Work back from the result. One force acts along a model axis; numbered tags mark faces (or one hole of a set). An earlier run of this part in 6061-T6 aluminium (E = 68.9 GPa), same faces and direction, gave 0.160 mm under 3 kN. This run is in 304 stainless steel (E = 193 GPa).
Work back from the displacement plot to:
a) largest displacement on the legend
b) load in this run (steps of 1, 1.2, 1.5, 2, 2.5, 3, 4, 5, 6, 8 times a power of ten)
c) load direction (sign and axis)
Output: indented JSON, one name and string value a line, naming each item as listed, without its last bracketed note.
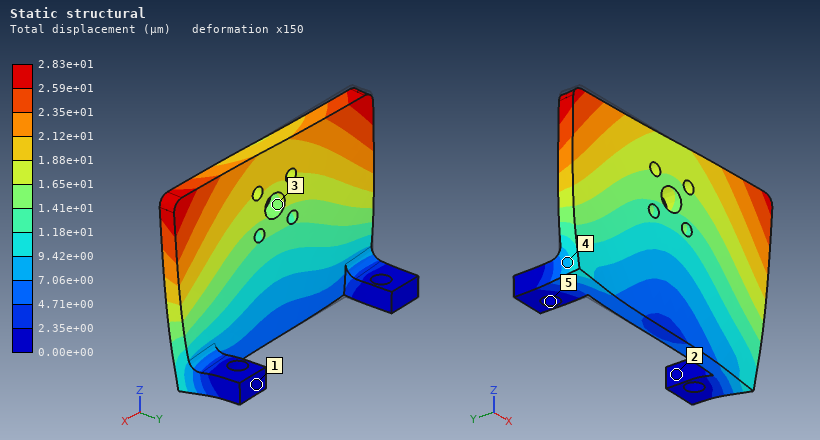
{
  "largest displacement on the legend": "2.83e+01 µm",
  "load in this run": "1.5 kN",
  "load direction": "+X"
}
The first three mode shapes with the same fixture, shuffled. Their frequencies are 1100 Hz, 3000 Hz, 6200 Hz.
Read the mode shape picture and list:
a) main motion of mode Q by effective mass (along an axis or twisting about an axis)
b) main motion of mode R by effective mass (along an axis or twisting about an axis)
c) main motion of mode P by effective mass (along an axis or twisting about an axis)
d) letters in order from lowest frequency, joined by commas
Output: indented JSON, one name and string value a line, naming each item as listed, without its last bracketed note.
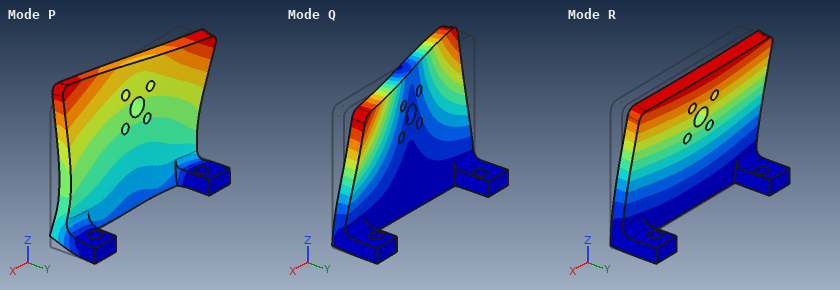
{
  "main motion of mode Q by effective mass": "twisting about Z",
  "main motion of mode R by effective mass": "along Y",
  "main motion of mode P by effective mass": "along X",
  "letters in order from lowest frequency, joined by commas": "R, Q, P"
}
